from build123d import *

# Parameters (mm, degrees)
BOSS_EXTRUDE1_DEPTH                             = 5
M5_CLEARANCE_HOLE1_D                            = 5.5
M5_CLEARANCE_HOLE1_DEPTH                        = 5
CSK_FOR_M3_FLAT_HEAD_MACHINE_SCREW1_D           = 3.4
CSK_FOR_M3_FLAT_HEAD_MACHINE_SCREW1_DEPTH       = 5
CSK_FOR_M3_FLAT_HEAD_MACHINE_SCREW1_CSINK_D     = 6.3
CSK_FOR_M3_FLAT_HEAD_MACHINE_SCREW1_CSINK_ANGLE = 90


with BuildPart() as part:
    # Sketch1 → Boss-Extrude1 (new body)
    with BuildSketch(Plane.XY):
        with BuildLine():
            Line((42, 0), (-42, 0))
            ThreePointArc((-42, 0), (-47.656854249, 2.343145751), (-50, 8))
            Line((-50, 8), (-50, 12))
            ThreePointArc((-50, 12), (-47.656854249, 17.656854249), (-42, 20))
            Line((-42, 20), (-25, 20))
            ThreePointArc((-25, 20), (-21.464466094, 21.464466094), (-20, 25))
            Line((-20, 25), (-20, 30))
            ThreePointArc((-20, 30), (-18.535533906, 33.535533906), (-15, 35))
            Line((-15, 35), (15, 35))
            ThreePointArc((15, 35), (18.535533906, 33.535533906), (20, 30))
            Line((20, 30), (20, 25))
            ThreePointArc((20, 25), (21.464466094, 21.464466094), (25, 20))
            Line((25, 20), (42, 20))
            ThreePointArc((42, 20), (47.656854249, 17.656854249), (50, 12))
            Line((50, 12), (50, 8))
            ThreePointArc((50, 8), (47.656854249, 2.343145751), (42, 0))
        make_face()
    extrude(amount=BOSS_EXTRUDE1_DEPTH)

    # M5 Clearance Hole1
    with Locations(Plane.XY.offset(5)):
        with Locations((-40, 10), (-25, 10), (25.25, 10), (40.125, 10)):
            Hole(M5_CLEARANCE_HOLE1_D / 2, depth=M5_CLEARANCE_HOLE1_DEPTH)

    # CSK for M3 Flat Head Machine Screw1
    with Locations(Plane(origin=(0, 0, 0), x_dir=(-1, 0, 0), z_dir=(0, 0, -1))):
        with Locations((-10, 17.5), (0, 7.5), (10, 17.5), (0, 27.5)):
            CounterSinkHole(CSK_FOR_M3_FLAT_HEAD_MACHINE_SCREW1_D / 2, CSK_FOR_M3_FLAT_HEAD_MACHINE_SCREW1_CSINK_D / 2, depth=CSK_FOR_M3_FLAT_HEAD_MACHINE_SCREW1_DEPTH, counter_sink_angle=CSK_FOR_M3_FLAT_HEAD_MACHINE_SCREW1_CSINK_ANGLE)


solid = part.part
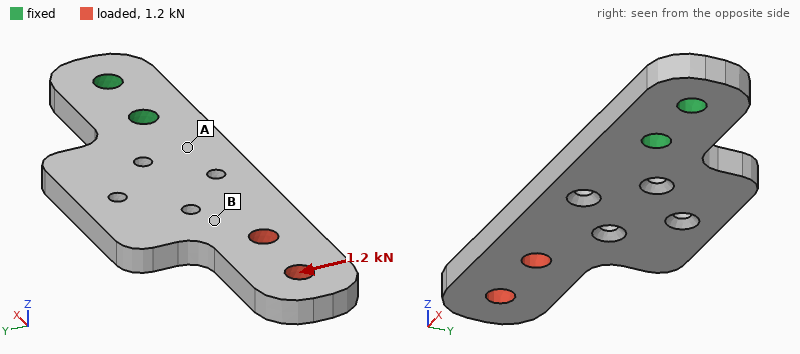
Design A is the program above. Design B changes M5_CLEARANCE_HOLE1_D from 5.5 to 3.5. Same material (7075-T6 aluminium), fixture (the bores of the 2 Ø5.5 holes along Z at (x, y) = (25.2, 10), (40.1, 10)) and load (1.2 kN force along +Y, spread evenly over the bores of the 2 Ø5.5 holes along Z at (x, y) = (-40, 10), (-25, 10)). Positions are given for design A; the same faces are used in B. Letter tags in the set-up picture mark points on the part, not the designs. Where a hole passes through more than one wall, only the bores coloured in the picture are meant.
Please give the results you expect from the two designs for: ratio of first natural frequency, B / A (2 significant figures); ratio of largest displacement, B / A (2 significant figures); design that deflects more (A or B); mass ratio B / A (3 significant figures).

0.94
1.1
B
1.02
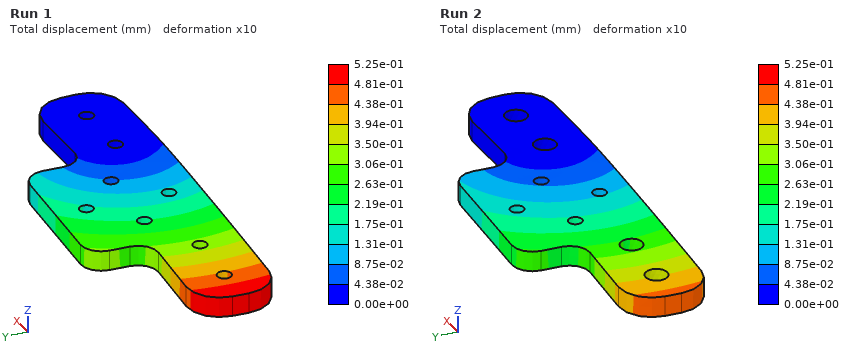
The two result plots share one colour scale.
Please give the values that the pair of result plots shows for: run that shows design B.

Run 1
